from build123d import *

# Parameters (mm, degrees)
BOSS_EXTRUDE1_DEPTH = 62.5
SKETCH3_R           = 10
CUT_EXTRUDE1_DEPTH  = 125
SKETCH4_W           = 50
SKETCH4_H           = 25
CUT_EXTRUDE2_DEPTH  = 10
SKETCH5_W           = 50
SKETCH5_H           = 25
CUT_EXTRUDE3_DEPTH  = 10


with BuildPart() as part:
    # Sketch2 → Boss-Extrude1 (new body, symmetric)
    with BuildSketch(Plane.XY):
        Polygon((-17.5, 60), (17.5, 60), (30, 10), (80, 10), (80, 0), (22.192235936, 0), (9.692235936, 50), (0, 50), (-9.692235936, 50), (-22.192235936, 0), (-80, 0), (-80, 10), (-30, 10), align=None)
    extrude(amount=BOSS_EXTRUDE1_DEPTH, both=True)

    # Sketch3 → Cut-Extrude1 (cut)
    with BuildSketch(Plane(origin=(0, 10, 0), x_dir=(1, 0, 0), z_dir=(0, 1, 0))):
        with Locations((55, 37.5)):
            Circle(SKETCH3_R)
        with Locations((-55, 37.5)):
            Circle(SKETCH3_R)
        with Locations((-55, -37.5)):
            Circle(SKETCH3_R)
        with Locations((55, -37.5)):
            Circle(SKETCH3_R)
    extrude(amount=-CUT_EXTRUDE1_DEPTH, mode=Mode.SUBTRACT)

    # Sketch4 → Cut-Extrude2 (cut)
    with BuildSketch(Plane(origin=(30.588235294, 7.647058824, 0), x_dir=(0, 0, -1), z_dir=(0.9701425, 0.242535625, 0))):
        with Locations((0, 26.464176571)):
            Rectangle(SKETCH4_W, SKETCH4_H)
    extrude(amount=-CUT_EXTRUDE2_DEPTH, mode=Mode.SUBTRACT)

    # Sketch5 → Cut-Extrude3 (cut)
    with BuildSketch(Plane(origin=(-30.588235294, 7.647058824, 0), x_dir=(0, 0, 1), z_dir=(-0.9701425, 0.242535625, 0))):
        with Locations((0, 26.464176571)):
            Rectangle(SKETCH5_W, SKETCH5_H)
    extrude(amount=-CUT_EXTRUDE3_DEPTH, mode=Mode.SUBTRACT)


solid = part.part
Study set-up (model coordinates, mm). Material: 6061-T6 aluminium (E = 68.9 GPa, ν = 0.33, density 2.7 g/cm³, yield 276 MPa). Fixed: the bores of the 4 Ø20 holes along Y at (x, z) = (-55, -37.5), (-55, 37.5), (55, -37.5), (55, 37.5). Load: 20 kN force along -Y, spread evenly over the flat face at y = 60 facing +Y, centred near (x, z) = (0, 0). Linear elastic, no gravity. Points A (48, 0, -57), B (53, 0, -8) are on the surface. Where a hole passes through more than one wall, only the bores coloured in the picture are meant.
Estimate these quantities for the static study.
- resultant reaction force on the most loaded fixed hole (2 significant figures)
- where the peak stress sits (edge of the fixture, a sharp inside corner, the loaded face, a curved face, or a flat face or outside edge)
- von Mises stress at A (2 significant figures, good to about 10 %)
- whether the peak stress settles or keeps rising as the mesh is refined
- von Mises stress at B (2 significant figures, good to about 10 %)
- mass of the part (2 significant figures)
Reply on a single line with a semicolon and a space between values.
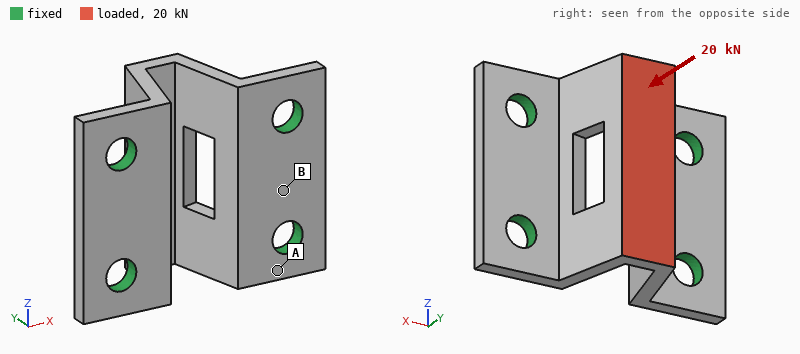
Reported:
5.5 kN; edge of the fixture; 34 MPa; keeps rising; 15 MPa; 700 g
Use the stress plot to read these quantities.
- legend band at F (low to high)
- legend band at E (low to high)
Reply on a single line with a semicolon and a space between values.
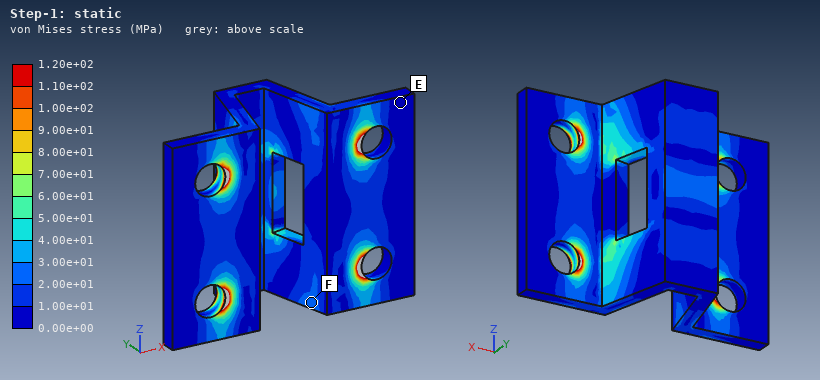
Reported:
2.00e+01 to 3.00e+01 MPa; 0.00e+00 to 1.00e+01 MPa
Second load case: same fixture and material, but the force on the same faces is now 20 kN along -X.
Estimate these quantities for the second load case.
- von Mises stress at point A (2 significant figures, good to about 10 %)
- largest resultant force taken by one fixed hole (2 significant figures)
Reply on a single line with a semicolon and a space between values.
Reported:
31 MPa; 8.7 kN
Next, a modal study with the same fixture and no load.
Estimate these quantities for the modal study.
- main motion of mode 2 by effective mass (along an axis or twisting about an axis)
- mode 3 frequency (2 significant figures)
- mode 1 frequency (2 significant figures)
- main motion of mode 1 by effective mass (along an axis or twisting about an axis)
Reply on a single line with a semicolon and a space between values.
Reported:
along X; 4700 Hz; 3400 Hz; along Z
